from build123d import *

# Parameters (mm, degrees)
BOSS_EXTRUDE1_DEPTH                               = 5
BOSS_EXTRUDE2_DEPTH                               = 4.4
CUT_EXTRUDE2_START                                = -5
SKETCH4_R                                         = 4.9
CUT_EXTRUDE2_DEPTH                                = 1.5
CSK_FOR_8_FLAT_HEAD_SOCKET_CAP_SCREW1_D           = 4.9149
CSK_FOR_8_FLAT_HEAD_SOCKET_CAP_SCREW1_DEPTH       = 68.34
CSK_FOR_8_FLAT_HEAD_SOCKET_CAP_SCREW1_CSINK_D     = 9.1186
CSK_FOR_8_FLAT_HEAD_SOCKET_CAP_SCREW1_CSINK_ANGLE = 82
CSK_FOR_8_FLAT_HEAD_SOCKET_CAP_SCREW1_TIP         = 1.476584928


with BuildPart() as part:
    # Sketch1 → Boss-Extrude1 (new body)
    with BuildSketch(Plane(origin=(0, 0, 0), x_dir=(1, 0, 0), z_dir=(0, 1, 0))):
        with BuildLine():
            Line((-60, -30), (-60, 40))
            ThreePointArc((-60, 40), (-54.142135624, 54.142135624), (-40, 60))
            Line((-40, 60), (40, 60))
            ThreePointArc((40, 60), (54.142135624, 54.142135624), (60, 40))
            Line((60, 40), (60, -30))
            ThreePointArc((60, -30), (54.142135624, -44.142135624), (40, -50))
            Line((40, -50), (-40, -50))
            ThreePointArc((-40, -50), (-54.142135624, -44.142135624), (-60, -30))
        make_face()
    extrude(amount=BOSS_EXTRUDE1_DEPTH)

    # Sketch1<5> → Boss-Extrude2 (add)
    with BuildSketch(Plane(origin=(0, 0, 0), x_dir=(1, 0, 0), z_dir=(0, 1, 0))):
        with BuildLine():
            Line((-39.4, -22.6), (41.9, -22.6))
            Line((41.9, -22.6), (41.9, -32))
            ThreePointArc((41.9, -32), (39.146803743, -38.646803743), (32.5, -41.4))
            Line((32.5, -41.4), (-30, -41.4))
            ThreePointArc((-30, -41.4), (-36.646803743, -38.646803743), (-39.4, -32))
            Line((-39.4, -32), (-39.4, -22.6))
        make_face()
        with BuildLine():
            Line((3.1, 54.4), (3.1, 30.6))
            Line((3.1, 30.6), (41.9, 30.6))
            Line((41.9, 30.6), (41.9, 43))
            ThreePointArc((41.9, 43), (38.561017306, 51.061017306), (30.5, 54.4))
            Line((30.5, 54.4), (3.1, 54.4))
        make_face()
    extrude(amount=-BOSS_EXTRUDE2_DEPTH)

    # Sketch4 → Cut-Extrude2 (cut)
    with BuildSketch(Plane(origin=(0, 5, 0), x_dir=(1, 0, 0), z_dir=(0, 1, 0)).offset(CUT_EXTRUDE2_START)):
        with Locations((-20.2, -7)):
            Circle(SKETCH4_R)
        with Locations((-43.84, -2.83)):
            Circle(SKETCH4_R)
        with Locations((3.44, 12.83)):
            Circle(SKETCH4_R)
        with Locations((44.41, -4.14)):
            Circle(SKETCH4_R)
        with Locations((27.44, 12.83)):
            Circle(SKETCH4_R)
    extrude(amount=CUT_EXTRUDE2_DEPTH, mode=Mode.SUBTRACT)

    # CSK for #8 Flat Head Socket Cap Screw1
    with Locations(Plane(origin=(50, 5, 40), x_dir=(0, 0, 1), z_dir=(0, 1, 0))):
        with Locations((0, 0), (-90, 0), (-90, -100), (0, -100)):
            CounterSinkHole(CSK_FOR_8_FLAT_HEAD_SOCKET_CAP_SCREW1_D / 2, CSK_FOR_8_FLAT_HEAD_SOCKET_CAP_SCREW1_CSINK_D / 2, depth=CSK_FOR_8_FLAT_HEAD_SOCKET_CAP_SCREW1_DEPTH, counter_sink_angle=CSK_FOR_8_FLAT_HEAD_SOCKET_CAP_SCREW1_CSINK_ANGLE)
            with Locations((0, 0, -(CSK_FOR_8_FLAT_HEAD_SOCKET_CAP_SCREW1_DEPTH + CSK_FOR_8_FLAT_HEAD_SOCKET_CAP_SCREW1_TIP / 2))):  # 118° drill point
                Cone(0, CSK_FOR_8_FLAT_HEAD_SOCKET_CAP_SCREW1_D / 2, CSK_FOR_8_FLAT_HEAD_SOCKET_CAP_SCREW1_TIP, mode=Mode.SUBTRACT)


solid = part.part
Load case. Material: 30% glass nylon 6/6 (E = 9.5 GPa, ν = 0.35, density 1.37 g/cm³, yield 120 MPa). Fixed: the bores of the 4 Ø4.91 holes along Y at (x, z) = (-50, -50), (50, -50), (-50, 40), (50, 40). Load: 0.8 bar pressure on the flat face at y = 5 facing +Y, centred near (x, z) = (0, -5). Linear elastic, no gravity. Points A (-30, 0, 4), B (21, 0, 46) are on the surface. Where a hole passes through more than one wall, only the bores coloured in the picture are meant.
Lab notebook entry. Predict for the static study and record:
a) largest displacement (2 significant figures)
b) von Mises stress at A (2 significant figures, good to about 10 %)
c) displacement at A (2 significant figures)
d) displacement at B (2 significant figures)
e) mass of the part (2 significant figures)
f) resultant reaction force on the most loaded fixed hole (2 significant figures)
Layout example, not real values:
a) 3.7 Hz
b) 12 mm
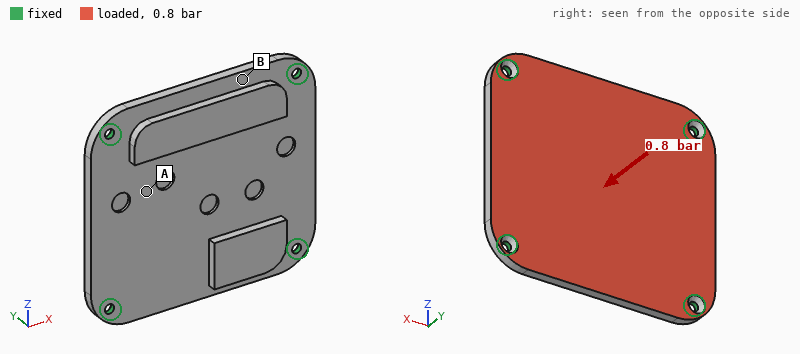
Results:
a) 0.50 mm
b) 9.2 MPa
c) 0.38 mm
d) 0.11 mm
e) 100 g
f) 350 N
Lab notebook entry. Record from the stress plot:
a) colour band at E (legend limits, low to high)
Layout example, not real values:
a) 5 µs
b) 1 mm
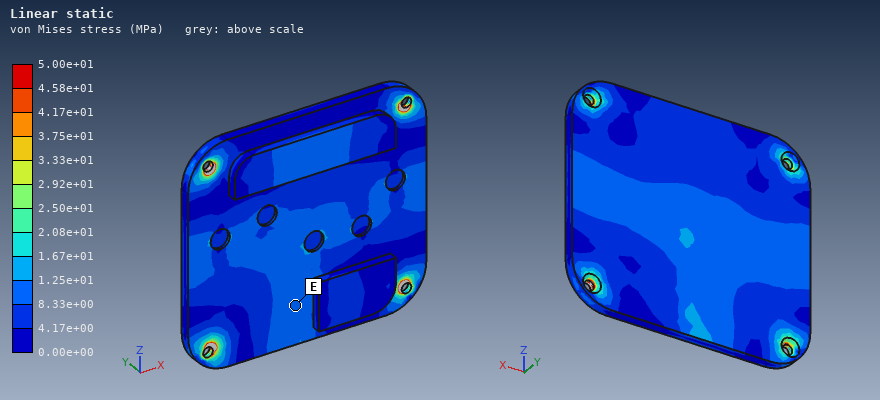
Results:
a) 8.33e+00 to 1.25e+01 MPa
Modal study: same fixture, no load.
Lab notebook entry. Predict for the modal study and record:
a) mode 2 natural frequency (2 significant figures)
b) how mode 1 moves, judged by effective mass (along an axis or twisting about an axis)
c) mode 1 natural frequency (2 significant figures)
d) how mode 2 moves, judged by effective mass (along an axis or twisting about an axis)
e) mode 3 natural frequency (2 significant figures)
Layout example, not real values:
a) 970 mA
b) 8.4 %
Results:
a) 1400 Hz
b) along Y
c) 900 Hz
d) twisting about X
e) 1700 Hz
